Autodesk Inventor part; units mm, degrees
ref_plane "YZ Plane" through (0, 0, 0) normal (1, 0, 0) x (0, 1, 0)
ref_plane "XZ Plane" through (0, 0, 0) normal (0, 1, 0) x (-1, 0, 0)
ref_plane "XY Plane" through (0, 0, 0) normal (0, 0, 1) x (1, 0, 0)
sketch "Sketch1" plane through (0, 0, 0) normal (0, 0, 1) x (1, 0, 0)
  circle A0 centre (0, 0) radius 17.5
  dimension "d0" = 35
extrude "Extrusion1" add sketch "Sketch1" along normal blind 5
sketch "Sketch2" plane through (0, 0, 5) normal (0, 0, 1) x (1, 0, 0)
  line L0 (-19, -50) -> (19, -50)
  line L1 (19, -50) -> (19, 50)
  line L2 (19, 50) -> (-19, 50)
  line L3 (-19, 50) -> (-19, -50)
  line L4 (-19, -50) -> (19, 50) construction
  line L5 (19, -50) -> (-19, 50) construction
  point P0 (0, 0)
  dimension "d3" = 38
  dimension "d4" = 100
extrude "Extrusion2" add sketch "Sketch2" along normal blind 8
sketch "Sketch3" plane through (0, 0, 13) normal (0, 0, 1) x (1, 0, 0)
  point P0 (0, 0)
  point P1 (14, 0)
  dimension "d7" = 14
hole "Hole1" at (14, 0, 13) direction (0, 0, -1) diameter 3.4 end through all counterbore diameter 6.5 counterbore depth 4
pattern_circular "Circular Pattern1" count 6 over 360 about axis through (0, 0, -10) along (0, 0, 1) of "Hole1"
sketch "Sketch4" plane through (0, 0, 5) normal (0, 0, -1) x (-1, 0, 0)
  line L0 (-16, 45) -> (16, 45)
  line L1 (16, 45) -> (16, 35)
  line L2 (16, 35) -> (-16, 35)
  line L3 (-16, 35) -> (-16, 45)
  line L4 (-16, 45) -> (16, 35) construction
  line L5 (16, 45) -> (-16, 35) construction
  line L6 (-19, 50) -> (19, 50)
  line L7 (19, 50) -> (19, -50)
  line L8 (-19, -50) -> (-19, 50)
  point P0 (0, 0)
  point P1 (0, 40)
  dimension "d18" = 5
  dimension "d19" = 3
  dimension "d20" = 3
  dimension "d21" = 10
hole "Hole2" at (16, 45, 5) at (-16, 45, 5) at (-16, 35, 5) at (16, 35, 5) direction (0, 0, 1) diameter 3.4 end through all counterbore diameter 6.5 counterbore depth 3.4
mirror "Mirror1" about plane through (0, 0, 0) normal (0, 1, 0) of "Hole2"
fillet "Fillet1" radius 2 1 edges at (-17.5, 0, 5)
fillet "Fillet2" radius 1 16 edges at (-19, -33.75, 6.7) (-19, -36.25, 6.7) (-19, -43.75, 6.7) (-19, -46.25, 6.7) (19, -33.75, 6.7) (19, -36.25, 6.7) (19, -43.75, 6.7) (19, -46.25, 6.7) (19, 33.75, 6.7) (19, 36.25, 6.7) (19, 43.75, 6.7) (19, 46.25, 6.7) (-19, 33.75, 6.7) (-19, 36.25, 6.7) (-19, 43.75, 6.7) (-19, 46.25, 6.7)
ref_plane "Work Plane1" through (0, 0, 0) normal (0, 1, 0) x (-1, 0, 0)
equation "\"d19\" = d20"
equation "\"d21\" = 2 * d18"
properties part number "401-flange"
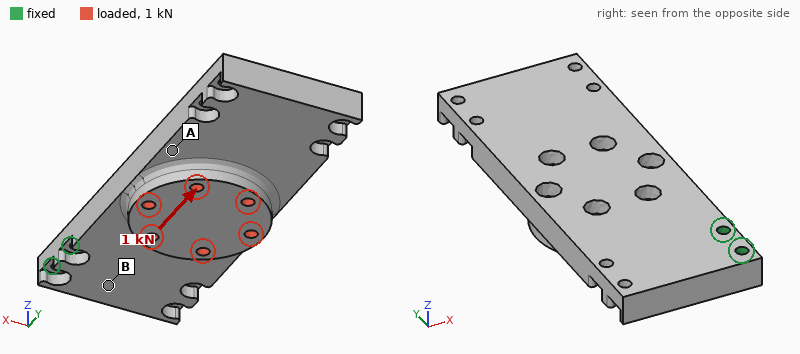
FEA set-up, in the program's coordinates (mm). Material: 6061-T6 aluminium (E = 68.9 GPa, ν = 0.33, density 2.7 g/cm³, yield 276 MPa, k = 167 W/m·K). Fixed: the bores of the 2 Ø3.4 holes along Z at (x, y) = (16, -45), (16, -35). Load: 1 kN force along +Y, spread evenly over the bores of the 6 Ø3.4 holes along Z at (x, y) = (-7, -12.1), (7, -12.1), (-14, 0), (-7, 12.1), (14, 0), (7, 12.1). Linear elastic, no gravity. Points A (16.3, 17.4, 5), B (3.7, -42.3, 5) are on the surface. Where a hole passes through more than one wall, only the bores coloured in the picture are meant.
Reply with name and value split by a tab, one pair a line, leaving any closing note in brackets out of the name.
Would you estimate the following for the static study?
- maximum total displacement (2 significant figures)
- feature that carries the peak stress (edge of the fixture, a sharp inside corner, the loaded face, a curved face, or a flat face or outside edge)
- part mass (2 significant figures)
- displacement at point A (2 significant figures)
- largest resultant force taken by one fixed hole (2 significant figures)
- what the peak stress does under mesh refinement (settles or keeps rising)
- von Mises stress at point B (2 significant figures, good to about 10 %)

maximum total displacement	0.15 mm
feature that carries the peak stress	edge of the fixture
part mass	88 g
displacement at point A	0.083 mm
largest resultant force taken by one fixed hole	1.4 kN
what the peak stress does under mesh refinement	keeps rising
von Mises stress at point B	18 MPa
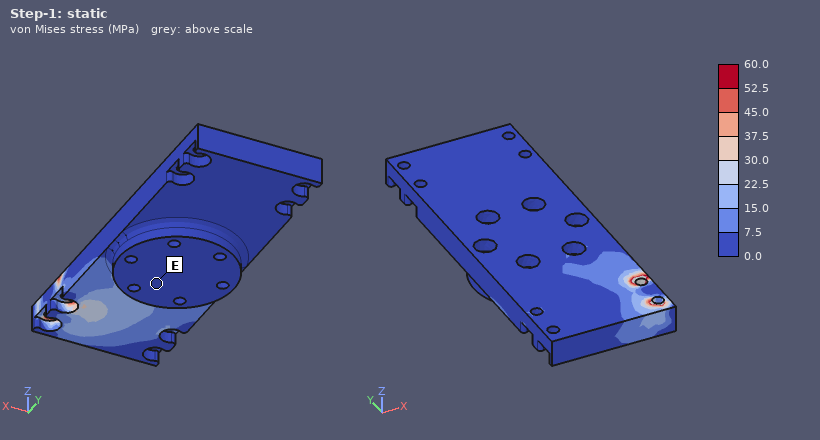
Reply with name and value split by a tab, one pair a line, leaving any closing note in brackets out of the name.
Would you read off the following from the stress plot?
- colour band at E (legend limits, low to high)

colour band at E	0.0 to 7.5 MPa
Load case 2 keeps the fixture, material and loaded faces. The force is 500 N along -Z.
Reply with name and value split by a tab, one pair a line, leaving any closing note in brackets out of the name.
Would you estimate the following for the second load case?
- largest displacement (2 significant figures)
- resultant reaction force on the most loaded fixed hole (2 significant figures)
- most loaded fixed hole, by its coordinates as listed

largest displacement	0.57 mm
resultant reaction force on the most loaded fixed hole	1.5 kN
most loaded fixed hole, by its coordinates as listed	(16, -35)
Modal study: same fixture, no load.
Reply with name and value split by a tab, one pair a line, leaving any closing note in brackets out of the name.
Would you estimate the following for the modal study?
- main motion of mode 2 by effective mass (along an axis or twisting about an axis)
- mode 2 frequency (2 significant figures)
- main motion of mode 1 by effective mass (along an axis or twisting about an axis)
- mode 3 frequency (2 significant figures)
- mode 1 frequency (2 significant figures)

main motion of mode 2 by effective mass	along X
mode 2 frequency	1500 Hz
main motion of mode 1 by effective mass	along Z
mode 3 frequency	2100 Hz
mode 1 frequency	630 Hz
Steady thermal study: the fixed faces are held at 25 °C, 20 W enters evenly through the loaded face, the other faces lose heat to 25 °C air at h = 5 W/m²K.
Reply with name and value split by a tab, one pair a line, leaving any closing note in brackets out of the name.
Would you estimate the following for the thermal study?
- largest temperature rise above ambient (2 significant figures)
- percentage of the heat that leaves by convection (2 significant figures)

largest temperature rise above ambient	20 K
percentage of the heat that leaves by convection	4.2 %
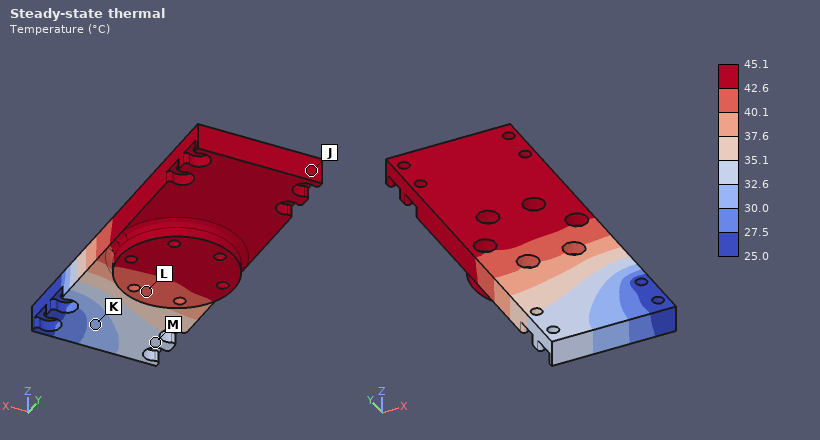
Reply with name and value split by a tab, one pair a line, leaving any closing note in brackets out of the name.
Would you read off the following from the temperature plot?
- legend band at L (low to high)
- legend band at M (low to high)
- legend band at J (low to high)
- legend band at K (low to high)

legend band at L	40.1 to 42.6 °C
legend band at M	32.6 to 35.1 °C
legend band at J	42.6 to 45.1 °C
legend band at K	30.0 to 32.6 °C
